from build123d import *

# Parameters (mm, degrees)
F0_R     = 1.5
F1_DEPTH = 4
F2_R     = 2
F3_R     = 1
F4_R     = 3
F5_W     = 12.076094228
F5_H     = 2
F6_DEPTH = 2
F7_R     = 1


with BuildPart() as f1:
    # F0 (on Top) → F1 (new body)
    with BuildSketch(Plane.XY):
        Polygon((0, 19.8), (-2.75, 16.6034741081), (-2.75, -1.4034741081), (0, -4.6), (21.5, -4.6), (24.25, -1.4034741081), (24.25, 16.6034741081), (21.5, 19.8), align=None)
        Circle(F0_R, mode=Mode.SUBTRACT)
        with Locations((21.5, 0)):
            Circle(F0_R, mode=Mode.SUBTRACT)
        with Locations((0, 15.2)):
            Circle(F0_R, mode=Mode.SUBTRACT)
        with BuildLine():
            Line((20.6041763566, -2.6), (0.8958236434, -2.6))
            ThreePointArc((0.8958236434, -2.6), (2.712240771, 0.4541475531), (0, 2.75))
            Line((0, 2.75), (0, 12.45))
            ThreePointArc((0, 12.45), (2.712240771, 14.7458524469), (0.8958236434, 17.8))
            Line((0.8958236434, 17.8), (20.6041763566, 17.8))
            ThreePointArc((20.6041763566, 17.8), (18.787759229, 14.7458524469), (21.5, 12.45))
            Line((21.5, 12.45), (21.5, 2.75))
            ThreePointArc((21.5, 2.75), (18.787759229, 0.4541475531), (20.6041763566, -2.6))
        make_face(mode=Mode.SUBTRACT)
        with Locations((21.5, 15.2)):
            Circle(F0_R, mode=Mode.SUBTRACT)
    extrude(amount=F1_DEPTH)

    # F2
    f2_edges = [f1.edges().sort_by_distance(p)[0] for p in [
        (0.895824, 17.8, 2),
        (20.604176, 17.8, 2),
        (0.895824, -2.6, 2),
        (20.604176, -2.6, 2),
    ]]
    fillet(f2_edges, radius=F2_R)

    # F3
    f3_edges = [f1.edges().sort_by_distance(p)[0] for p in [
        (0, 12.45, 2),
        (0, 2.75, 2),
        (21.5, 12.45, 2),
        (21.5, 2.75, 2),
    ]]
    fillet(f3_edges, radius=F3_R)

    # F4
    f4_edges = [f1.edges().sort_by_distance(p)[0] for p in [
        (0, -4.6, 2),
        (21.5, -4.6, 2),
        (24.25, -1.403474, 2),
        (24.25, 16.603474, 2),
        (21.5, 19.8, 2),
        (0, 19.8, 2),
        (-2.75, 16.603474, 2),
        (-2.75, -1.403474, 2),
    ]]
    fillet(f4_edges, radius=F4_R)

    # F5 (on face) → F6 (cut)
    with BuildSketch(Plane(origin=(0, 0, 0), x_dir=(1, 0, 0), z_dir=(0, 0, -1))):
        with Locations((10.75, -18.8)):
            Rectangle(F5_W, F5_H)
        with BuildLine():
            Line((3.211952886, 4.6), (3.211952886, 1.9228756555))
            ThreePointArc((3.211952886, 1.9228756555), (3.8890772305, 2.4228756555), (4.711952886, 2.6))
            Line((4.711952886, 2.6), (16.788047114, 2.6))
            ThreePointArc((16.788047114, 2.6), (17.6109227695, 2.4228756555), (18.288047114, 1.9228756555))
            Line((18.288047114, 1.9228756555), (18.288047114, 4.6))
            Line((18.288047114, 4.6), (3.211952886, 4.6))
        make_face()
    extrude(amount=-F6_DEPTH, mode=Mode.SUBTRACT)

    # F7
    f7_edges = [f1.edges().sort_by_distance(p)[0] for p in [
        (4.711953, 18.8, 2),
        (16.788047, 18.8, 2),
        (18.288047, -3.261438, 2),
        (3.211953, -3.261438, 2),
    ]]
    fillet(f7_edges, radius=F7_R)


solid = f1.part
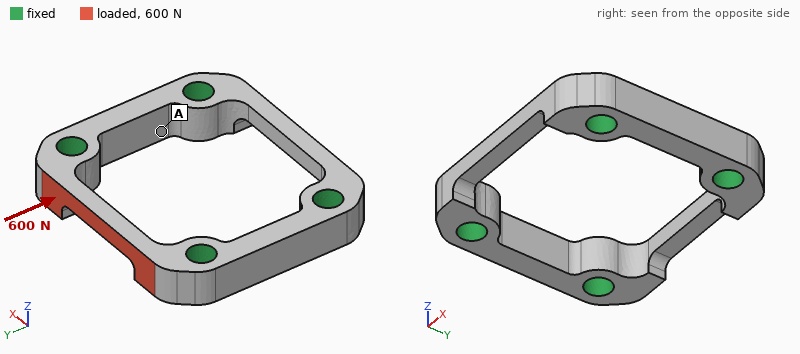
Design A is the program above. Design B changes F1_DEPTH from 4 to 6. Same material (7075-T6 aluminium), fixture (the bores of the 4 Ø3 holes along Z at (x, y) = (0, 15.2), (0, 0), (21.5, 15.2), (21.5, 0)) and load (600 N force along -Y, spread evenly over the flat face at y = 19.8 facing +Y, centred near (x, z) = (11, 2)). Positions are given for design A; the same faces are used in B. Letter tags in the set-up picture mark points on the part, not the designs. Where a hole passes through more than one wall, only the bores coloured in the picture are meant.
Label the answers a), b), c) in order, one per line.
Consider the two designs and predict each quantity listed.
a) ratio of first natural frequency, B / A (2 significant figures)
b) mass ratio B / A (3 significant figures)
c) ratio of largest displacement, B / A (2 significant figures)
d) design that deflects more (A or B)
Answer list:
a) 1.0
b) 1.57
c) 0.64
d) A
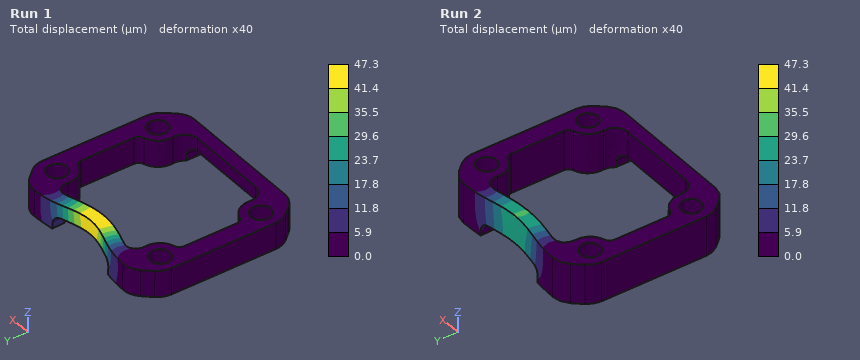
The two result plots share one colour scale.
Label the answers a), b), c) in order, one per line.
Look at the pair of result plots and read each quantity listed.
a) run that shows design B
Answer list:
a) Run 2
